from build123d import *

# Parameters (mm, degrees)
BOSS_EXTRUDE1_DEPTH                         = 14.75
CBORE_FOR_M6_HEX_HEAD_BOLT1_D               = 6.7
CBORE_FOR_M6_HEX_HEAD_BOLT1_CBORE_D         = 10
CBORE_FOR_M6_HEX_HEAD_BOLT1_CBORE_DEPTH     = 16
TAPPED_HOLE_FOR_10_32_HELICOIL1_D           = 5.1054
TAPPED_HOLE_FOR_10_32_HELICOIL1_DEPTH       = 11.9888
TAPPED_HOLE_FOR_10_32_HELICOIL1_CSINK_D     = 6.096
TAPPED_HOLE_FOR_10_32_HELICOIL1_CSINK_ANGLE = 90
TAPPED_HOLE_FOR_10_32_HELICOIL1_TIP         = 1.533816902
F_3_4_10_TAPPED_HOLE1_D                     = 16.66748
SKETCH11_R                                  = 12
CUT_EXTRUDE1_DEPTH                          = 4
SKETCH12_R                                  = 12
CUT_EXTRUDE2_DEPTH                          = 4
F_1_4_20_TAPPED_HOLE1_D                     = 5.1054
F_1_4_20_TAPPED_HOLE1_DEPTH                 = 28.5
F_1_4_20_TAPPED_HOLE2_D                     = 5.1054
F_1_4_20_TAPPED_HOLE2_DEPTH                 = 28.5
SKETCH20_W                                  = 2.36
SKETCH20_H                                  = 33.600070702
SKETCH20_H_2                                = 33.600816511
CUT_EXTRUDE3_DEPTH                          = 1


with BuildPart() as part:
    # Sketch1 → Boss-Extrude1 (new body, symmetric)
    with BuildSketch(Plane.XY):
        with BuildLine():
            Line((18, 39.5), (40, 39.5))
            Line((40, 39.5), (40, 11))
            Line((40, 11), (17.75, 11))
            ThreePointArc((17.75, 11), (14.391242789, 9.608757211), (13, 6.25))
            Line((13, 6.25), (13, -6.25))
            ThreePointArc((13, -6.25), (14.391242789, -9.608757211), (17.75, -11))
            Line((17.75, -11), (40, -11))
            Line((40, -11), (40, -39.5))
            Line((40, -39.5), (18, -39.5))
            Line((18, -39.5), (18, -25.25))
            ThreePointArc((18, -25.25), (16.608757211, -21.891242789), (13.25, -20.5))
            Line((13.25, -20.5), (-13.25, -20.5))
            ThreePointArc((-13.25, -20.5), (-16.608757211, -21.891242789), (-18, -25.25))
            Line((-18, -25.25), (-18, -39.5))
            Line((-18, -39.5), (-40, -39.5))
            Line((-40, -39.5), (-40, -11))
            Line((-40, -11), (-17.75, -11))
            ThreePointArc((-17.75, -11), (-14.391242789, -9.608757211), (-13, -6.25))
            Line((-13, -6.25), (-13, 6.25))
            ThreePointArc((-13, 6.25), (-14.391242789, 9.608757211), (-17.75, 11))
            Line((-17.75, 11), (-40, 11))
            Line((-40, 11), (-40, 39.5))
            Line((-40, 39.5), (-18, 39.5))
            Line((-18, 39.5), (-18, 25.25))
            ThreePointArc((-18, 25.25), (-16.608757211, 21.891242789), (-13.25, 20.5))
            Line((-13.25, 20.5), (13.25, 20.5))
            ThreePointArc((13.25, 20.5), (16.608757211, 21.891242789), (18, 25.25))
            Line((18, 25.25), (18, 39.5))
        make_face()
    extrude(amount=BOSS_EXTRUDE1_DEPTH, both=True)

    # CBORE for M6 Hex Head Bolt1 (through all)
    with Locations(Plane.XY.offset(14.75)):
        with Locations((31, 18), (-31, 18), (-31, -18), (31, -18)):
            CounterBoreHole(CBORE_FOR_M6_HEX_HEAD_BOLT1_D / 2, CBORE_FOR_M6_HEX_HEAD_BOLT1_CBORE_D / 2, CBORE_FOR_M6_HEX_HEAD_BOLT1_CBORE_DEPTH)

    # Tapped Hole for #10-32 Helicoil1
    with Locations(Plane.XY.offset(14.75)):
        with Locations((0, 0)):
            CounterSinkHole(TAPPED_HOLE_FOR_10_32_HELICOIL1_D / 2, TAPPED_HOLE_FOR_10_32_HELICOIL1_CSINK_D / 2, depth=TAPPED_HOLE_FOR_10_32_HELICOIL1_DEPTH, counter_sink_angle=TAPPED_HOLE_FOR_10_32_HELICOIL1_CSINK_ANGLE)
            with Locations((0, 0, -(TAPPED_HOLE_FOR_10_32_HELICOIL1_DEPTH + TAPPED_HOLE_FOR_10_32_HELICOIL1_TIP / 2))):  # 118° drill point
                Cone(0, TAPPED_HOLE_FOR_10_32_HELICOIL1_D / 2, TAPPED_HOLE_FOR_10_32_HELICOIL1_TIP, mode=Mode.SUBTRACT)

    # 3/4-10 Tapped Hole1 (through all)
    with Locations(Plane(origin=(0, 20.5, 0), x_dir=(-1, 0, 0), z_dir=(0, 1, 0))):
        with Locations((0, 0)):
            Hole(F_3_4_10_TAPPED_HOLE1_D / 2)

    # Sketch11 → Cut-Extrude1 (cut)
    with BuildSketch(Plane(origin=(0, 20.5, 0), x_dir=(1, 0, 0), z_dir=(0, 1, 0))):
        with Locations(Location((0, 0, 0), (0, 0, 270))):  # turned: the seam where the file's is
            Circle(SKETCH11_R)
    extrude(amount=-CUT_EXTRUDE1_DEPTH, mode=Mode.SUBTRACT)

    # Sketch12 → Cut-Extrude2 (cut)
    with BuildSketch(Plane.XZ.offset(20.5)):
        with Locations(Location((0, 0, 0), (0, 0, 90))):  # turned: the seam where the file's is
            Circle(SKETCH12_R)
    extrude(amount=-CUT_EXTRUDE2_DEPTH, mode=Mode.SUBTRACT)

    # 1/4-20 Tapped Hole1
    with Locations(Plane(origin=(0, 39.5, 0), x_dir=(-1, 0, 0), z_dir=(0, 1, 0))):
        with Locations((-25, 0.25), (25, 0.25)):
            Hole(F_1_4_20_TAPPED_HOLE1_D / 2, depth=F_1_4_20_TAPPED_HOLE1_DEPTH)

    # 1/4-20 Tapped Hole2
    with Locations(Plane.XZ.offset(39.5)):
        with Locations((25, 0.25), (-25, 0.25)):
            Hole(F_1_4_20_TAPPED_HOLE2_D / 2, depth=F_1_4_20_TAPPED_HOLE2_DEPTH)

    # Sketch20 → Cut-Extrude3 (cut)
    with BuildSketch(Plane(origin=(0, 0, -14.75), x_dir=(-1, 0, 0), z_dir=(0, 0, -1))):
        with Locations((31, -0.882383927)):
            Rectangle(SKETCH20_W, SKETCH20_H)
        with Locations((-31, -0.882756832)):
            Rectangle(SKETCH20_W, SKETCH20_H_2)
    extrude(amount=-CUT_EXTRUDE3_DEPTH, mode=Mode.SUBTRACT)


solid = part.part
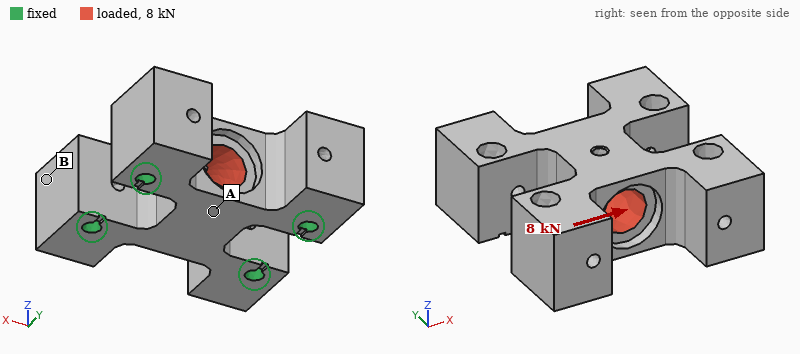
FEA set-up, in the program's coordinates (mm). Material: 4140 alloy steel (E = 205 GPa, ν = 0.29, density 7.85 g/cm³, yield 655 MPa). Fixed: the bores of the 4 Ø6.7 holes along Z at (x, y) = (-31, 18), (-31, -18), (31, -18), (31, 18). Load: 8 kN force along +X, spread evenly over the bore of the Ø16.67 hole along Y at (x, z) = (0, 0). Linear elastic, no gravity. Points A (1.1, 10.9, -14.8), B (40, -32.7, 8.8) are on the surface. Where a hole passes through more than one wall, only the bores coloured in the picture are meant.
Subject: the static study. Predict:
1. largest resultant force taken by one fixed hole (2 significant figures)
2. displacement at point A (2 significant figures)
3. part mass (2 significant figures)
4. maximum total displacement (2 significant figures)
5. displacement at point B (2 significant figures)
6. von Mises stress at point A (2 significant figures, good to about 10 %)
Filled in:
2.1 kN
1.3 µm
720 g
2.5 µm
1.2 µm
6.6 MPa
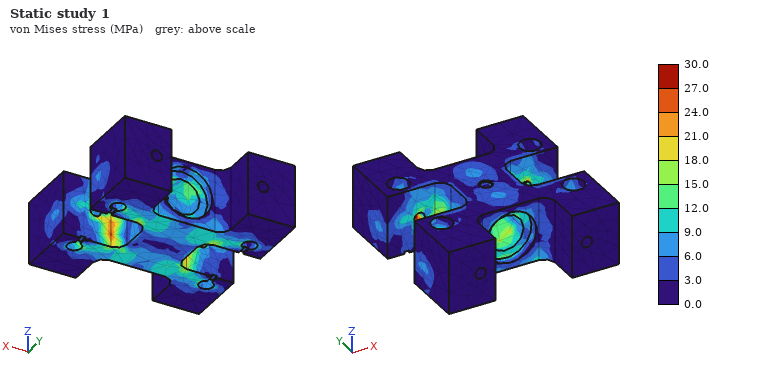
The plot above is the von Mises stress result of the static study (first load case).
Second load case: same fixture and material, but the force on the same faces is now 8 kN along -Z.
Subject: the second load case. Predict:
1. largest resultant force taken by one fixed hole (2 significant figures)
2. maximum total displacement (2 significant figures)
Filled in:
2.1 kN
4.9 µm
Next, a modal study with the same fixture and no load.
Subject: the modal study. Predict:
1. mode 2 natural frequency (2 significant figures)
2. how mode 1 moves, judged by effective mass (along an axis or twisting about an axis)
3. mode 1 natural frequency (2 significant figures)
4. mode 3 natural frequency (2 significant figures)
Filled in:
12 kHz
along Y
10000 Hz
12 kHz
